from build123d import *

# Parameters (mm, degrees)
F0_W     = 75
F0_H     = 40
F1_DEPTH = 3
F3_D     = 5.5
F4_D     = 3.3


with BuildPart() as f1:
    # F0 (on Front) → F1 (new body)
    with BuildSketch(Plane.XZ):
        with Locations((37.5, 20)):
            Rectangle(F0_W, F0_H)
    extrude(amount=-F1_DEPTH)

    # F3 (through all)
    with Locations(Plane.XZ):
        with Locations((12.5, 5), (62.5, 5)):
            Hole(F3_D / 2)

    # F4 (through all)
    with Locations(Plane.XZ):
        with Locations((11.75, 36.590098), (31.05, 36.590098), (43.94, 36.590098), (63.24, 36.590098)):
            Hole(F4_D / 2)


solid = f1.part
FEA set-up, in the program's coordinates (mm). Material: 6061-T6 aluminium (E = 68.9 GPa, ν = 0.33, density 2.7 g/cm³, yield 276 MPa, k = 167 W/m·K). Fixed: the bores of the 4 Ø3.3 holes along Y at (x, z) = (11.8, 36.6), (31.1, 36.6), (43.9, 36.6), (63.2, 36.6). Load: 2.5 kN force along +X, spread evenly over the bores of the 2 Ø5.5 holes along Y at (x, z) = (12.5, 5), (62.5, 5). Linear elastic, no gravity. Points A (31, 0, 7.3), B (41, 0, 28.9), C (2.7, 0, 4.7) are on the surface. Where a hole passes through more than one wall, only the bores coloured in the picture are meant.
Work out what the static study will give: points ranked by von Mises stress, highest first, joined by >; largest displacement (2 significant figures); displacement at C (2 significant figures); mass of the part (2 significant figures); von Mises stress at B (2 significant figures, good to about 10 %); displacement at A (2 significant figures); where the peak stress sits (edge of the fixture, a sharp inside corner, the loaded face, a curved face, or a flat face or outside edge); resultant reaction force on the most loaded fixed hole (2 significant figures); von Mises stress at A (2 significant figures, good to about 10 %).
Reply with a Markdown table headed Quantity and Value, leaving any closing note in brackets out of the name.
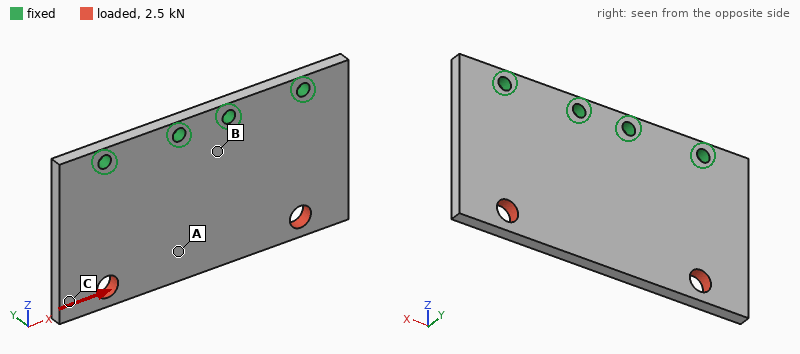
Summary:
| Quantity | Value |
|---|---|
| points ranked by von Mises stress, highest first, joined by > | B > A > C |
| largest displacement | 39 µm |
| displacement at C | 34 µm |
| mass of the part | 24 g |
| von Mises stress at B | 32 MPa |
| displacement at A | 22 µm |
| where the peak stress sits | edge of the fixture |
| resultant reaction force on the most loaded fixed hole | 1.5 kN |
| von Mises stress at A | 20 MPa |
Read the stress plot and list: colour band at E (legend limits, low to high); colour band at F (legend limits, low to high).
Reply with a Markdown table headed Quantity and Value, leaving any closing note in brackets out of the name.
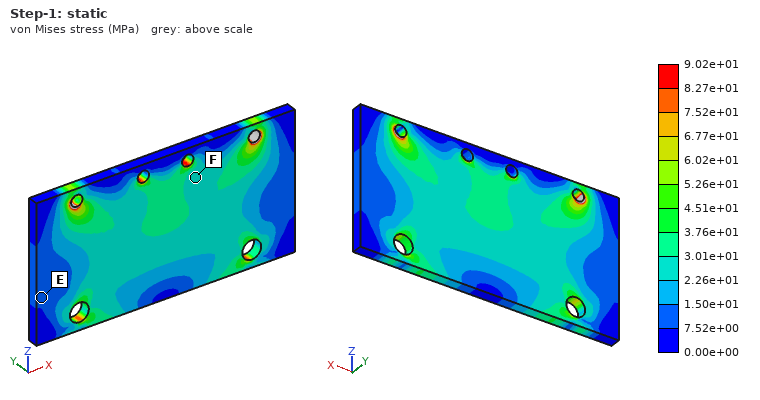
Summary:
| Quantity | Value |
|---|---|
| colour band at E | 7.52e+00 to 1.50e+01 MPa |
| colour band at F | 2.26e+01 to 3.01e+01 MPa |
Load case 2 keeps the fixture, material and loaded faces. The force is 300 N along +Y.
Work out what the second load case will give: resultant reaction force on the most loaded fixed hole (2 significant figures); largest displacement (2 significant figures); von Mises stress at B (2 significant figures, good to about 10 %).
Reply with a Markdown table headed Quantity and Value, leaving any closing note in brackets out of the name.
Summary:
| Quantity | Value |
|---|---|
| resultant reaction force on the most loaded fixed hole | 95 N |
| largest displacement | 0.36 mm |
| von Mises stress at B | 59 MPa |
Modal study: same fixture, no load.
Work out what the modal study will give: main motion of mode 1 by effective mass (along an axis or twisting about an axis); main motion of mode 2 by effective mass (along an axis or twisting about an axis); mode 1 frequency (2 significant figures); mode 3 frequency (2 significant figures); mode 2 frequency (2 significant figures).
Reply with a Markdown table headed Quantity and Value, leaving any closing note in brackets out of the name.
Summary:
| Quantity | Value |
|---|---|
| main motion of mode 1 by effective mass | along Y |
| main motion of mode 2 by effective mass | twisting about Z |
| mode 1 frequency | 1900 Hz |
| mode 3 frequency | 4900 Hz |
| mode 2 frequency | 2700 Hz |
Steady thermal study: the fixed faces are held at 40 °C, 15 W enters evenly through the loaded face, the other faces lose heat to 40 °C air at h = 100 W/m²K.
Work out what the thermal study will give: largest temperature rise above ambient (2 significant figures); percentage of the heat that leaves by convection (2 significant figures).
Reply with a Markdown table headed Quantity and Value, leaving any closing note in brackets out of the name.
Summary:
| Quantity | Value |
|---|---|
| largest temperature rise above ambient | 16 K |
| percentage of the heat that leaves by convection | 25 % |
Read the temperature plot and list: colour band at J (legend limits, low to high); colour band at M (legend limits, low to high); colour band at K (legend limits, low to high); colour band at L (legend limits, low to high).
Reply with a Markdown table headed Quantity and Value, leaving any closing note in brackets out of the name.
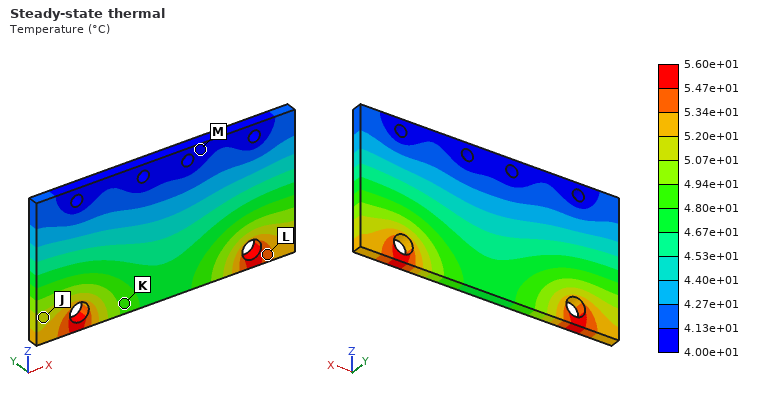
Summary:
| Quantity | Value |
|---|---|
| colour band at J | 5.07e+01 to 5.20e+01 °C |
| colour band at M | 4.00e+01 to 4.13e+01 °C |
| colour band at K | 4.80e+01 to 4.94e+01 °C |
| colour band at L | 5.34e+01 to 5.47e+01 °C |
